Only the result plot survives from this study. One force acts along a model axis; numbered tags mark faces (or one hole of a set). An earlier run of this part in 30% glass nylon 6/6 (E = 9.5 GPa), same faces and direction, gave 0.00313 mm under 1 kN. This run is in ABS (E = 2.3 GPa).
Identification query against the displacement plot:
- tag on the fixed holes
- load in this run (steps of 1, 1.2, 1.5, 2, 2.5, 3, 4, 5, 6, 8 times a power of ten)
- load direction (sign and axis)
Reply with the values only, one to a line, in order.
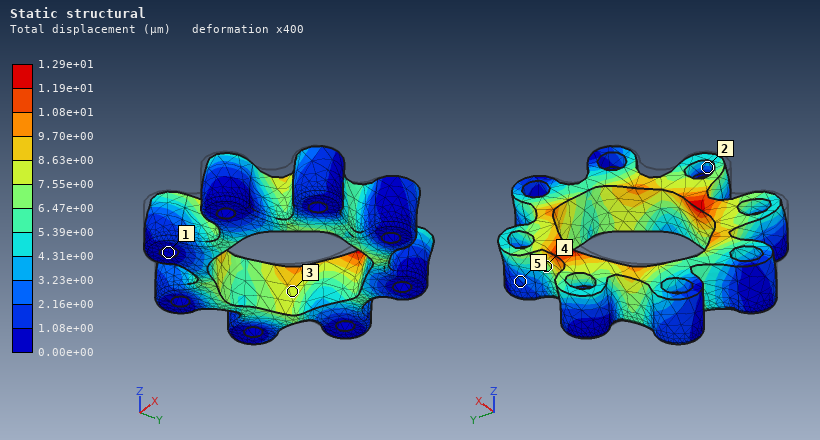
1
1 kN
+Y
